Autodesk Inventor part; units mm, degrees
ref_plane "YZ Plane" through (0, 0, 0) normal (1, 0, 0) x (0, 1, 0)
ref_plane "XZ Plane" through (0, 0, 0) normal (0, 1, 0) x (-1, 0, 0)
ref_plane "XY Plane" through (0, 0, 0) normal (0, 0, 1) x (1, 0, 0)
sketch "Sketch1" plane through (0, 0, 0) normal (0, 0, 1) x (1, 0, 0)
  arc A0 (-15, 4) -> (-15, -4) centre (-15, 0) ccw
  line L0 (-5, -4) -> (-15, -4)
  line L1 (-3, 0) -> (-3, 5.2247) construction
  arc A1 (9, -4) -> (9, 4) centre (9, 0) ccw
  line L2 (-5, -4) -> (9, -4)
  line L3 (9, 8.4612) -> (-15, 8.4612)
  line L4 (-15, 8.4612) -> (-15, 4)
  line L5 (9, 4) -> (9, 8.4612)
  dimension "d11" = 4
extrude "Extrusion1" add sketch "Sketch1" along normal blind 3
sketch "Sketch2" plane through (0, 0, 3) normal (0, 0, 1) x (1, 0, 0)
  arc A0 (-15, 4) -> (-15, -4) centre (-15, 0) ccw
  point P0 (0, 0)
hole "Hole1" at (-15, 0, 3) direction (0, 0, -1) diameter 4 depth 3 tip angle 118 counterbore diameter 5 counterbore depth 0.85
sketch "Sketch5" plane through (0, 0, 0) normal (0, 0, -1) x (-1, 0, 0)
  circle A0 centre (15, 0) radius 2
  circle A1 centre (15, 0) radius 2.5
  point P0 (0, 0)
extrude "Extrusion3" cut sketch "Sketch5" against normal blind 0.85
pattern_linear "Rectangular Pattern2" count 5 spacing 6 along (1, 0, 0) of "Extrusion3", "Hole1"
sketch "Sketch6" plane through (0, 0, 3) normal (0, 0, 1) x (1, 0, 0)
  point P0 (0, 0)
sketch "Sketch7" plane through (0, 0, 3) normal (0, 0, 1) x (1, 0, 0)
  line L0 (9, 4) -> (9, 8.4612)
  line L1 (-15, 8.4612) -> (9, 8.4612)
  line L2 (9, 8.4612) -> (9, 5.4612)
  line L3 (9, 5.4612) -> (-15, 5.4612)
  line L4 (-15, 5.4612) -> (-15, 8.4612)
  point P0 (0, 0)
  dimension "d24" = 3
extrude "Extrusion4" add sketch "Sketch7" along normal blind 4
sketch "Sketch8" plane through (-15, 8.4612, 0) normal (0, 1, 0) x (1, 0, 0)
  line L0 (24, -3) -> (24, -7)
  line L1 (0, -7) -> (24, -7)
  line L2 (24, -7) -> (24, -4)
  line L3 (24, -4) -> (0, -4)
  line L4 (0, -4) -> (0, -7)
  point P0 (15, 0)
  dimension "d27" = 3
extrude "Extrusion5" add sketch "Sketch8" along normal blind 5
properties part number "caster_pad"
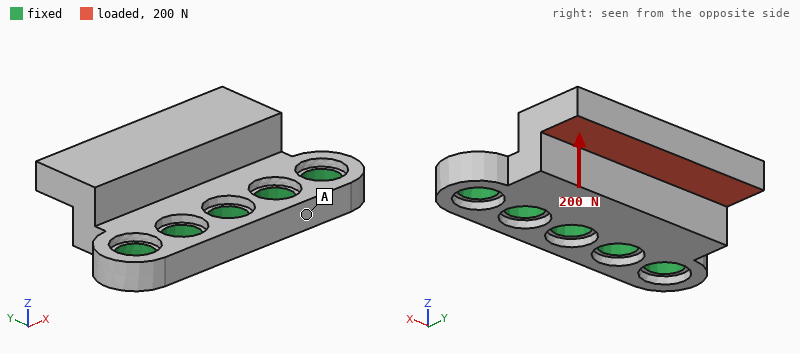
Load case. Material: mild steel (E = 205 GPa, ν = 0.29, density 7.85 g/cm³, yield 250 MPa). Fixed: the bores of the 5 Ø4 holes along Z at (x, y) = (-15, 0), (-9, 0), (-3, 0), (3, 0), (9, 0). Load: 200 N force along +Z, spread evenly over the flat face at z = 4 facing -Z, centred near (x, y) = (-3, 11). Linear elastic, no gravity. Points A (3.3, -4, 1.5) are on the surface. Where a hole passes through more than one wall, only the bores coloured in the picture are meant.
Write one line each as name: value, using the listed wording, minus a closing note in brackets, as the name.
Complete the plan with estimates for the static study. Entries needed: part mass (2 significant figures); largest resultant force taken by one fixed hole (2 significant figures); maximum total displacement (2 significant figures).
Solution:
part mass: 11 g
largest resultant force taken by one fixed hole: 50 N
maximum total displacement: 17 µm
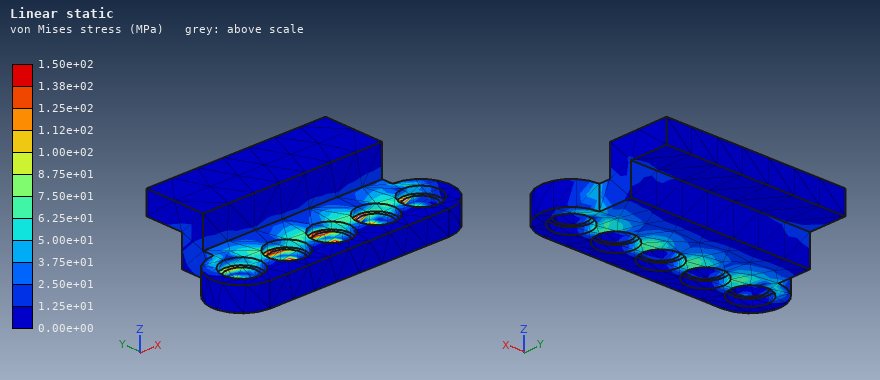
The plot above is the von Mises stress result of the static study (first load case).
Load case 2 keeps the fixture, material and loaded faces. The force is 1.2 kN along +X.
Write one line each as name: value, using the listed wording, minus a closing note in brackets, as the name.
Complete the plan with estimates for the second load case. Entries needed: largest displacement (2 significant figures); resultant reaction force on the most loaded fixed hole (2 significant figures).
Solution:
largest displacement: 8.2 µm
resultant reaction force on the most loaded fixed hole: 460 N
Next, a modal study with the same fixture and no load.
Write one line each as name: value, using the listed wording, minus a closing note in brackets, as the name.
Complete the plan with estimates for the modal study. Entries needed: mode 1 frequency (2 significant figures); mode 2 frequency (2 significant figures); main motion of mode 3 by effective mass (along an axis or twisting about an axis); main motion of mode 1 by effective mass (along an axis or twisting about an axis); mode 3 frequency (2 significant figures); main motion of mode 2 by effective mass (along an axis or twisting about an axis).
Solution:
mode 1 frequency: 9500 Hz
mode 2 frequency: 20 kHz
main motion of mode 3 by effective mass: along X
main motion of mode 1 by effective mass: along Z
mode 3 frequency: 40 kHz
main motion of mode 2 by effective mass: twisting about Y
